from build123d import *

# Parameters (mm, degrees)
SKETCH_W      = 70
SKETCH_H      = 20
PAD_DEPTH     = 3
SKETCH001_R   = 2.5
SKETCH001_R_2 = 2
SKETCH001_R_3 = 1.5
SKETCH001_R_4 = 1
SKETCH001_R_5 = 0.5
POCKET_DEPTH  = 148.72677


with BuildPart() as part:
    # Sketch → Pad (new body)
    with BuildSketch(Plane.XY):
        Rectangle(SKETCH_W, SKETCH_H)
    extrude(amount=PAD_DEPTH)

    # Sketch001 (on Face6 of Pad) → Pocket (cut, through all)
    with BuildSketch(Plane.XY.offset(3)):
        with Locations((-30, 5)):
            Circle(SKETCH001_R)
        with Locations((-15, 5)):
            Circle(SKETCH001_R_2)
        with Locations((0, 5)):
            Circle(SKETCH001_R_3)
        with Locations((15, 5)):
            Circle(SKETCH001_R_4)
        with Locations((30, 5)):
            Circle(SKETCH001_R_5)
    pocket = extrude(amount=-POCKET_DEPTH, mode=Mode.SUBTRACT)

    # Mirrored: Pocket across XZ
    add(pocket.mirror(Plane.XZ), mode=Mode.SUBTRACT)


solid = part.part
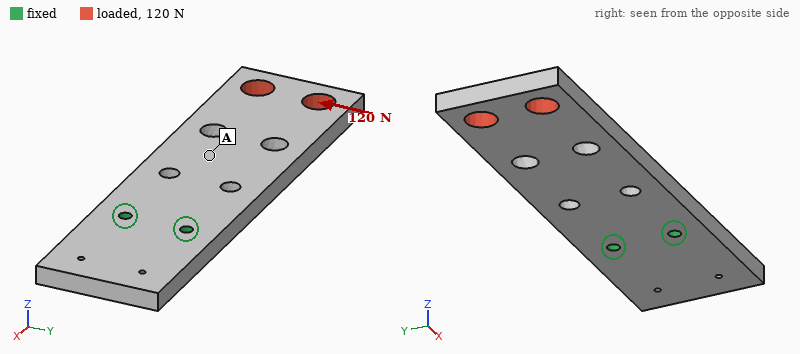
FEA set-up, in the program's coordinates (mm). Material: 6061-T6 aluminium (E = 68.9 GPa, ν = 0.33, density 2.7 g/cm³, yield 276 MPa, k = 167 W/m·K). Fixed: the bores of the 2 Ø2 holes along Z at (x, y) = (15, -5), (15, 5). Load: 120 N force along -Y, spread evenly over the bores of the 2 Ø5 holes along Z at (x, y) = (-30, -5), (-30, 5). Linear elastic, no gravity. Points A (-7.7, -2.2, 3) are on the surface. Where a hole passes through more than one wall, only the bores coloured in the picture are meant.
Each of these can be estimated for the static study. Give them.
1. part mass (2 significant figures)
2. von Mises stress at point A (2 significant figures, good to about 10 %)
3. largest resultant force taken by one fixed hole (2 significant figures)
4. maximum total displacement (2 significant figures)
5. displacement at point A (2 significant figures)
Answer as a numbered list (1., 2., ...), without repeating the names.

1. 11 g
2. 5.2 MPa
3. 490 N
4. 47 µm
5. 14 µm
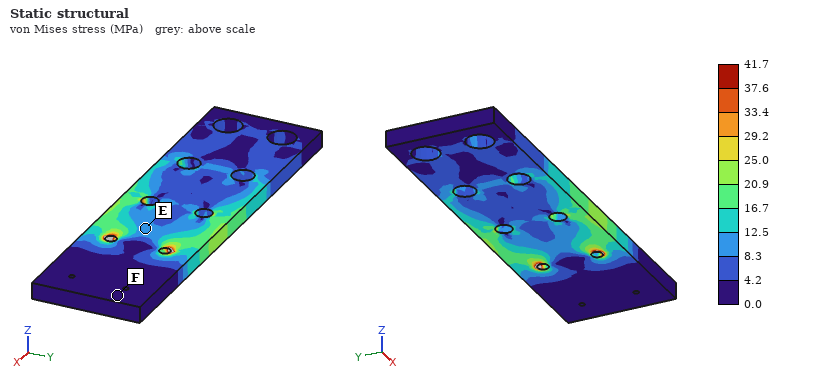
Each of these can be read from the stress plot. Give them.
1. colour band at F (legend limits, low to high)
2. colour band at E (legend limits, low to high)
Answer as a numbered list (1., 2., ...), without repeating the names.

1. 0.0 to 4.2 MPa
2. 8.3 to 12.5 MPa
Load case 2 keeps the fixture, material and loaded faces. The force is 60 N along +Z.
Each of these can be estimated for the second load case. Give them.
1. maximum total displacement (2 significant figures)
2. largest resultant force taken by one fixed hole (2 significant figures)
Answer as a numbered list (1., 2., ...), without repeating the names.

1. 0.74 mm
2. 30 N
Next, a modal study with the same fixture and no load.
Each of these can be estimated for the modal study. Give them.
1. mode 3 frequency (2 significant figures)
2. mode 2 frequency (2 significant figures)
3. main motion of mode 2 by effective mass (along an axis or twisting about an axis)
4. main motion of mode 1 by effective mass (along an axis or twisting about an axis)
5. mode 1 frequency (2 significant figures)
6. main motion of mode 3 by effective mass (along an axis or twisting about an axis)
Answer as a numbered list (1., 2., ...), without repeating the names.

1. 5400 Hz
2. 4800 Hz
3. twisting about X
4. along Z
5. 1000 Hz
6. along Y
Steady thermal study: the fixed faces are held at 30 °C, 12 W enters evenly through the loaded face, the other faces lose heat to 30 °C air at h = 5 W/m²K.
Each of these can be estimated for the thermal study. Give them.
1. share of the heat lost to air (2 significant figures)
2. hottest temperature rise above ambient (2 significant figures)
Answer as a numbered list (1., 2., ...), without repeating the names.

1. 3.2 %
2. 63 K
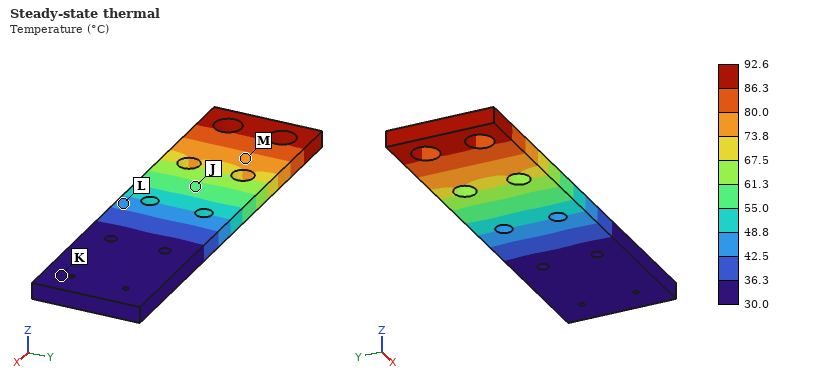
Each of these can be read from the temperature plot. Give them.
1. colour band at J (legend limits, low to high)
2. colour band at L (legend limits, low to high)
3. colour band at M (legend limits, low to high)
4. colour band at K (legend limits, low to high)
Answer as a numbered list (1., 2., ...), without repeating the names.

1. 55.0 to 61.3 °C
2. 42.5 to 48.8 °C
3. 73.8 to 80.0 °C
4. 30.0 to 36.3 °C
